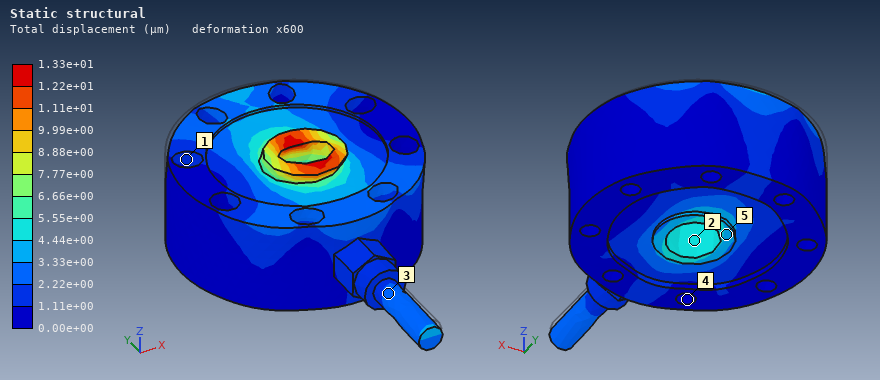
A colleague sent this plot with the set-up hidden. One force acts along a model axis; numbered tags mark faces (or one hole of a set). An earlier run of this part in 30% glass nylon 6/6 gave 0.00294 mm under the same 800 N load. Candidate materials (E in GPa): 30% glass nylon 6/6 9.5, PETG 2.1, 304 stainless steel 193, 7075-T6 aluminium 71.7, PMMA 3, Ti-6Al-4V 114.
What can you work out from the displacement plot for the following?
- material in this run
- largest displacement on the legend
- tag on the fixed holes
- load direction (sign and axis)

PETG
1.33e+01 µm
4
-Y
